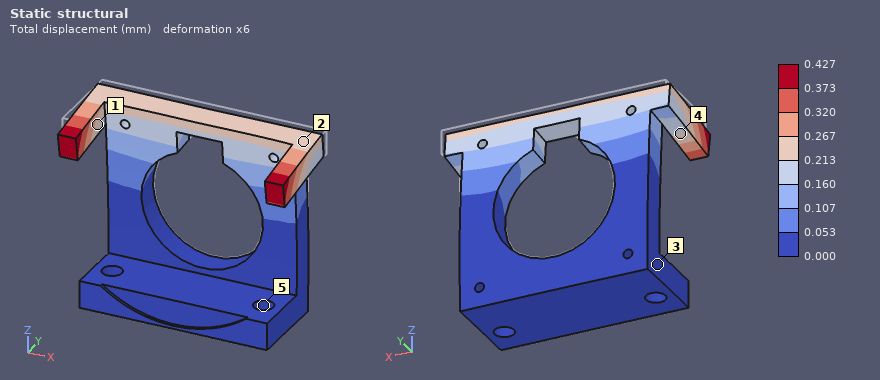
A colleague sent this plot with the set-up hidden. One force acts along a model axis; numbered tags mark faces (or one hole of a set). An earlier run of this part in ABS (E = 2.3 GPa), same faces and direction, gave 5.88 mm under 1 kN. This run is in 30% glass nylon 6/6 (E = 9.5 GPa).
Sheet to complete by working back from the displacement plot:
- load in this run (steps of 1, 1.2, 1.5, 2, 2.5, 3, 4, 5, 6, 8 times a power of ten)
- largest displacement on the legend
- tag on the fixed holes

300 N
0.427 mm
5
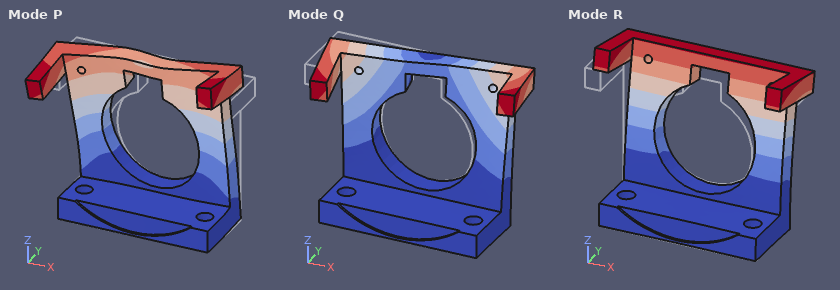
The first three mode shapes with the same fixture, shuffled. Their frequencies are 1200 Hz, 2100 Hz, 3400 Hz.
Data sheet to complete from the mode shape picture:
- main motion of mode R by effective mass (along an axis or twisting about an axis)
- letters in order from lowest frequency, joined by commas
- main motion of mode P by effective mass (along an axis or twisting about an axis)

along Y
R, Q, P
along X
